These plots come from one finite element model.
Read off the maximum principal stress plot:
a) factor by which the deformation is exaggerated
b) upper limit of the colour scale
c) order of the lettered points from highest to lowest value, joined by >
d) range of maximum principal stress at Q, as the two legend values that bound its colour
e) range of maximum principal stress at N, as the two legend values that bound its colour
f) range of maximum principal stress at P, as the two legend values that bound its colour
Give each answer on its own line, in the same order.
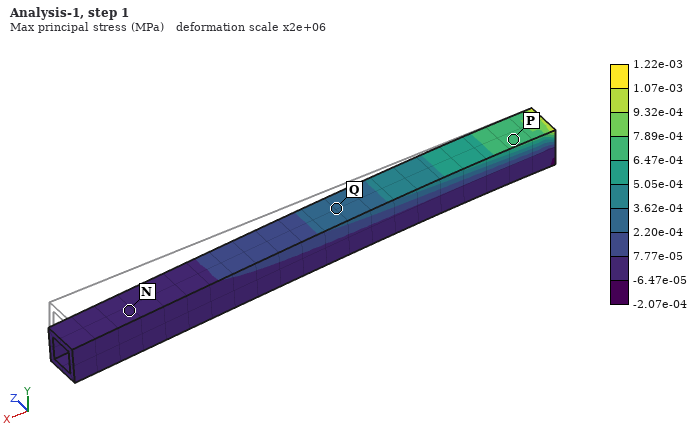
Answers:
2e+06
1.22e-03 MPa
P > Q > N
2.20e-04 to 3.62e-04 MPa
-6.47e-05 to 7.77e-05 MPa
6.47e-04 to 7.89e-04 MPa
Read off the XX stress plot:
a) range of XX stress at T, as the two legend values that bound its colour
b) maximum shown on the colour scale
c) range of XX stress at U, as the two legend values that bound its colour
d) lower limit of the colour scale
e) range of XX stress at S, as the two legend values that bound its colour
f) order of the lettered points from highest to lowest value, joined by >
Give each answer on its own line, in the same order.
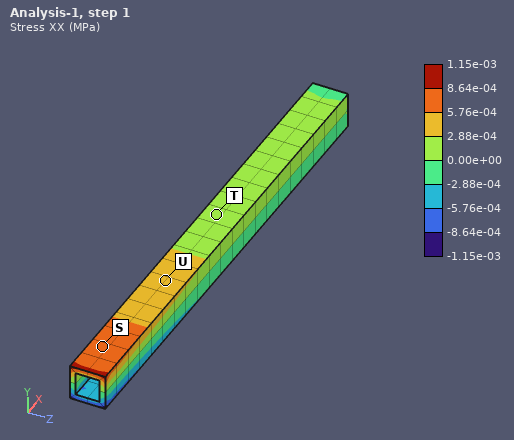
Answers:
0.00e+00 to 2.88e-04 MPa
1.15e-03 MPa
2.88e-04 to 5.76e-04 MPa
-1.15e-03 MPa
5.76e-04 to 8.64e-04 MPa
S > U > T
